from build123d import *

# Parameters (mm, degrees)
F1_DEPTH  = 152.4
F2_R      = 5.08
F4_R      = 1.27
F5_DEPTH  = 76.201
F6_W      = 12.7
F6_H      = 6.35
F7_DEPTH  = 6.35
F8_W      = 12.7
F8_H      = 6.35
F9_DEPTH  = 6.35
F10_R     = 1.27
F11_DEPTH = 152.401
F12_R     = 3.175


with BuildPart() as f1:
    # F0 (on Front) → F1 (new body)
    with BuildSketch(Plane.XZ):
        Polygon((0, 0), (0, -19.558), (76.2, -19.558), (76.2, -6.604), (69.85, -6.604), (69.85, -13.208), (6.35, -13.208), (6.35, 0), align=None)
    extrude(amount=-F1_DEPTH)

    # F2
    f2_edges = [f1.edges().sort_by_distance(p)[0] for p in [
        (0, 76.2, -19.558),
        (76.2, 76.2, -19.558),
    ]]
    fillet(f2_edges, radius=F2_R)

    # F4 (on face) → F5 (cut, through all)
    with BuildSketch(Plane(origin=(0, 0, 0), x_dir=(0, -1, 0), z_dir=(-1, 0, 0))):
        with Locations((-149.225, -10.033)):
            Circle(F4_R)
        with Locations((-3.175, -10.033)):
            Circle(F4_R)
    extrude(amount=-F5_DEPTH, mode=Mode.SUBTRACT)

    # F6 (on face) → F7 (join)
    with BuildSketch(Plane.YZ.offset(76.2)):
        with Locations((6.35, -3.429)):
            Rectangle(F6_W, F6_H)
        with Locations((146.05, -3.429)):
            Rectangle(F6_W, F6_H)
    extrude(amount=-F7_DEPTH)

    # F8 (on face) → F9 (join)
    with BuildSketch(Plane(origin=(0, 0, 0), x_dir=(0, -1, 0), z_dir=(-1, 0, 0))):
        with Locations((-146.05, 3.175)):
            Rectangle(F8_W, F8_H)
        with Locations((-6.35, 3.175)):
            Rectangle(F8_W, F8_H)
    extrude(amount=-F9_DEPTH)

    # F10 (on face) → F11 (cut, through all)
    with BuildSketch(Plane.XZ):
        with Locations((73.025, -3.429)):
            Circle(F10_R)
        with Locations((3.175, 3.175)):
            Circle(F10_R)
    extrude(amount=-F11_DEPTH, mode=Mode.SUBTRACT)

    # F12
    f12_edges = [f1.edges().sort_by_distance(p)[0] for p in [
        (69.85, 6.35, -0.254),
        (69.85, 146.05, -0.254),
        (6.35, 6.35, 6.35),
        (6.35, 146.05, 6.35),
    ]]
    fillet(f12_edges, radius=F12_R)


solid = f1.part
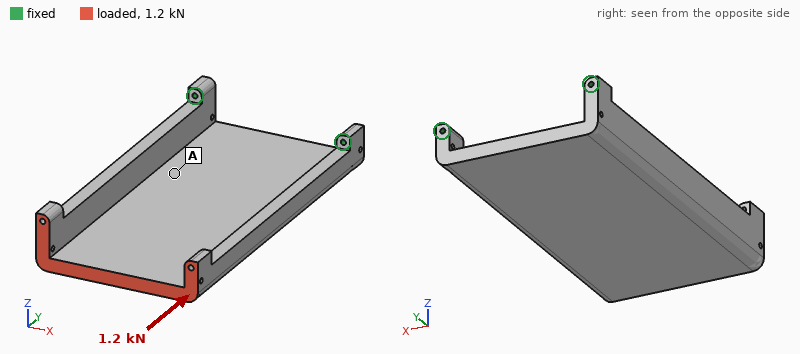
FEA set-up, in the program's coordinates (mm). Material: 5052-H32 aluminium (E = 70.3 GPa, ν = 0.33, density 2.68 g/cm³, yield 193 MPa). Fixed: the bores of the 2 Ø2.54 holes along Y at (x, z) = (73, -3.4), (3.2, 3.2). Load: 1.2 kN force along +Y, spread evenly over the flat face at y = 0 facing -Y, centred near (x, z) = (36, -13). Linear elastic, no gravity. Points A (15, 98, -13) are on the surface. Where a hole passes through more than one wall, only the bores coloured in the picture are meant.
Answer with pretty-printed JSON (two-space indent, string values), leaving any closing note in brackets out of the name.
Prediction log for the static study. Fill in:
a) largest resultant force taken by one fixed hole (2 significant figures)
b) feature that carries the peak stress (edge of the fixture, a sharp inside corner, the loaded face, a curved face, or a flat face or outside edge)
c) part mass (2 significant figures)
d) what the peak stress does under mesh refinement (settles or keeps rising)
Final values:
{
  "largest resultant force taken by one fixed hole": "630 N",
  "feature that carries the peak stress": "edge of the fixture",
  "part mass": "250 g",
  "what the peak stress does under mesh refinement": "keeps rising"
}
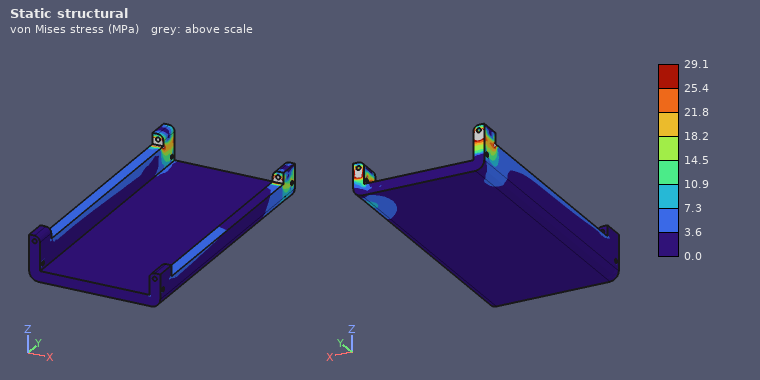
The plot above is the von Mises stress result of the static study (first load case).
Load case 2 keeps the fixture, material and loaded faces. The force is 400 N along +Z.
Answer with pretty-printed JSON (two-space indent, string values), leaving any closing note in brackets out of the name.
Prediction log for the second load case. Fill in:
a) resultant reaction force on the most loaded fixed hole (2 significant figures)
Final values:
{
  "resultant reaction force on the most loaded fixed hole": "210 N"
}
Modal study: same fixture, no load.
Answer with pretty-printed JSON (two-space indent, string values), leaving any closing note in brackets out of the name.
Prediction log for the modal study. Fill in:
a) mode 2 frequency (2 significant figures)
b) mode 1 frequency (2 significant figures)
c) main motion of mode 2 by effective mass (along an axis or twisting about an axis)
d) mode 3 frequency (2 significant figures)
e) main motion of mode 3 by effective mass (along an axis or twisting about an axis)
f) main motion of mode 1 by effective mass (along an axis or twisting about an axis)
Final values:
{
  "mode 2 frequency": "860 Hz",
  "mode 1 frequency": "340 Hz",
  "main motion of mode 2 by effective mass": "along X",
  "mode 3 frequency": "1700 Hz",
  "main motion of mode 3 by effective mass": "along X",
  "main motion of mode 1 by effective mass": "along Z"
}
